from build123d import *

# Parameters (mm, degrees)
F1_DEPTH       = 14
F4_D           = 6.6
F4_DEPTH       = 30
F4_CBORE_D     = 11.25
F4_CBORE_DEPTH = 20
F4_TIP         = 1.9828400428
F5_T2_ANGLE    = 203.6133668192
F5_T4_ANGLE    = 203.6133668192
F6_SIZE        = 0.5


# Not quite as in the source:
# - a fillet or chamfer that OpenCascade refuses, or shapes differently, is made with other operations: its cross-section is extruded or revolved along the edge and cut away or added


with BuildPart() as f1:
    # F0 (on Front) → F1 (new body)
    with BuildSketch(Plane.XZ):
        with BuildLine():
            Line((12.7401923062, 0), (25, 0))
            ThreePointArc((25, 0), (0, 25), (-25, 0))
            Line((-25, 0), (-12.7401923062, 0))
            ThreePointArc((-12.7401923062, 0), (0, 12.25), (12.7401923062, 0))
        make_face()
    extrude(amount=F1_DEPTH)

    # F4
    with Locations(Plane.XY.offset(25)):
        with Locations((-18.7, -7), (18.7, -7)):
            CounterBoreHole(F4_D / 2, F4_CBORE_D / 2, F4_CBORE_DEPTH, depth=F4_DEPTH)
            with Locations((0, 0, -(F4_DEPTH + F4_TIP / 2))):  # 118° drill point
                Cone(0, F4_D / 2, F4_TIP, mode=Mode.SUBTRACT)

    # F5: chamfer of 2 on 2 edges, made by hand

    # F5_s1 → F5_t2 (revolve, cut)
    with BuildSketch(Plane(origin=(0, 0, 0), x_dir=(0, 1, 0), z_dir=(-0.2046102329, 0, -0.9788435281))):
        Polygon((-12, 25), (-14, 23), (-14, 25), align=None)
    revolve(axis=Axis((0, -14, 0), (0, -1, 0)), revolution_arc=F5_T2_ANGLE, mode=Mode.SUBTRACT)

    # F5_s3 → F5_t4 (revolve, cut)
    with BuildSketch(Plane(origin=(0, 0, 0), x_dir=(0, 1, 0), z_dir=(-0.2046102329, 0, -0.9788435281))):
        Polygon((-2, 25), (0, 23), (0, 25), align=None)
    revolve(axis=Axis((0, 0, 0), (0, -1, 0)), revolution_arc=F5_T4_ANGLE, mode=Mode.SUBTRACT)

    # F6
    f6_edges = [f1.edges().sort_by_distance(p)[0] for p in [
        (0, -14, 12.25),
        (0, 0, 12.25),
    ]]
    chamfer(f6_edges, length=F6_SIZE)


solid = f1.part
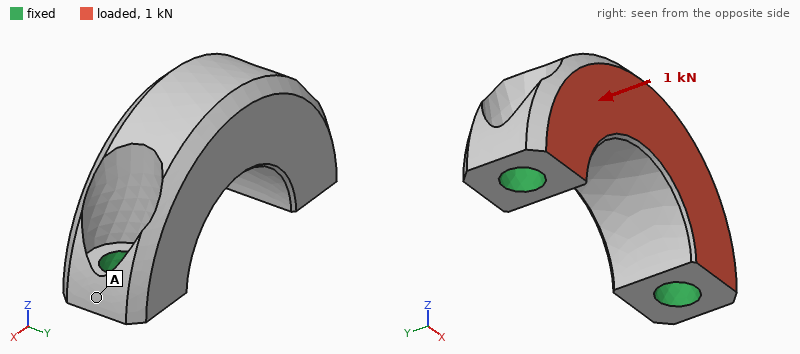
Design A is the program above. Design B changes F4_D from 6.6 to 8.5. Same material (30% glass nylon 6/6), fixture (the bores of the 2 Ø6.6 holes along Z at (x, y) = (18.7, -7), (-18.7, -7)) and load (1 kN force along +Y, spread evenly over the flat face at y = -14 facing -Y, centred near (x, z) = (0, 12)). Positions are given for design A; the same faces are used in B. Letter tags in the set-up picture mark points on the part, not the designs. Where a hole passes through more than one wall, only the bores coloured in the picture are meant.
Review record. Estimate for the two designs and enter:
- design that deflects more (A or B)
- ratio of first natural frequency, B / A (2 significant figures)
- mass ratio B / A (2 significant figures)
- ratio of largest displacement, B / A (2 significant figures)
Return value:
A
1.2
0.97
0.75
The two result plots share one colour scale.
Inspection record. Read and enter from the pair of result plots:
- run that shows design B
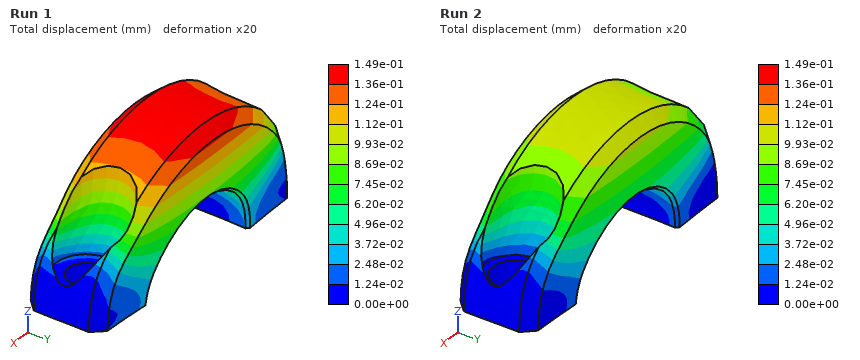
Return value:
Run 2
